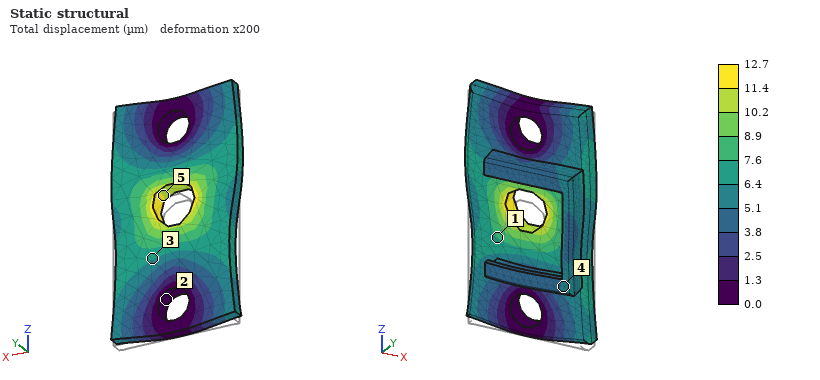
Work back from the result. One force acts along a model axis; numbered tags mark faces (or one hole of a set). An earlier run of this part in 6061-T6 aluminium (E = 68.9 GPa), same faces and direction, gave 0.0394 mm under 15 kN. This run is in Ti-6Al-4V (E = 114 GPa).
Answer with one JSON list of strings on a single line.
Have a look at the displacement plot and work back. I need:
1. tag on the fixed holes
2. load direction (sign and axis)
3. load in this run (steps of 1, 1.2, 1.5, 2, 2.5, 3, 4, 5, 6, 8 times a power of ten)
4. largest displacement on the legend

["2", "+Z", "8 kN", "12.7 µm"]
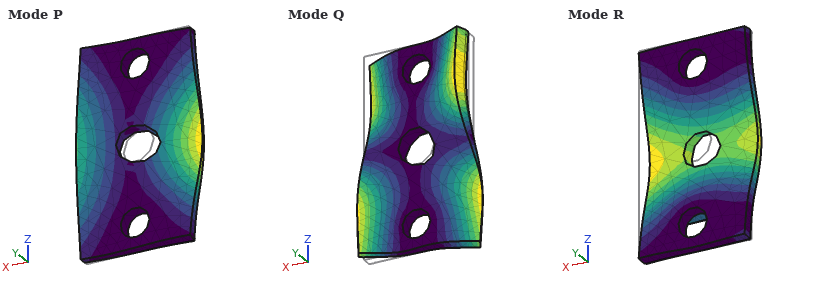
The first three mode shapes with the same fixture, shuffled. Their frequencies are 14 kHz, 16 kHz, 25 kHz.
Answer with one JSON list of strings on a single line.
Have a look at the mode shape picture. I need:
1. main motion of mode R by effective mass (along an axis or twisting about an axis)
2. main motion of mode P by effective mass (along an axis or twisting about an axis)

["along Y", "twisting about Z"]
